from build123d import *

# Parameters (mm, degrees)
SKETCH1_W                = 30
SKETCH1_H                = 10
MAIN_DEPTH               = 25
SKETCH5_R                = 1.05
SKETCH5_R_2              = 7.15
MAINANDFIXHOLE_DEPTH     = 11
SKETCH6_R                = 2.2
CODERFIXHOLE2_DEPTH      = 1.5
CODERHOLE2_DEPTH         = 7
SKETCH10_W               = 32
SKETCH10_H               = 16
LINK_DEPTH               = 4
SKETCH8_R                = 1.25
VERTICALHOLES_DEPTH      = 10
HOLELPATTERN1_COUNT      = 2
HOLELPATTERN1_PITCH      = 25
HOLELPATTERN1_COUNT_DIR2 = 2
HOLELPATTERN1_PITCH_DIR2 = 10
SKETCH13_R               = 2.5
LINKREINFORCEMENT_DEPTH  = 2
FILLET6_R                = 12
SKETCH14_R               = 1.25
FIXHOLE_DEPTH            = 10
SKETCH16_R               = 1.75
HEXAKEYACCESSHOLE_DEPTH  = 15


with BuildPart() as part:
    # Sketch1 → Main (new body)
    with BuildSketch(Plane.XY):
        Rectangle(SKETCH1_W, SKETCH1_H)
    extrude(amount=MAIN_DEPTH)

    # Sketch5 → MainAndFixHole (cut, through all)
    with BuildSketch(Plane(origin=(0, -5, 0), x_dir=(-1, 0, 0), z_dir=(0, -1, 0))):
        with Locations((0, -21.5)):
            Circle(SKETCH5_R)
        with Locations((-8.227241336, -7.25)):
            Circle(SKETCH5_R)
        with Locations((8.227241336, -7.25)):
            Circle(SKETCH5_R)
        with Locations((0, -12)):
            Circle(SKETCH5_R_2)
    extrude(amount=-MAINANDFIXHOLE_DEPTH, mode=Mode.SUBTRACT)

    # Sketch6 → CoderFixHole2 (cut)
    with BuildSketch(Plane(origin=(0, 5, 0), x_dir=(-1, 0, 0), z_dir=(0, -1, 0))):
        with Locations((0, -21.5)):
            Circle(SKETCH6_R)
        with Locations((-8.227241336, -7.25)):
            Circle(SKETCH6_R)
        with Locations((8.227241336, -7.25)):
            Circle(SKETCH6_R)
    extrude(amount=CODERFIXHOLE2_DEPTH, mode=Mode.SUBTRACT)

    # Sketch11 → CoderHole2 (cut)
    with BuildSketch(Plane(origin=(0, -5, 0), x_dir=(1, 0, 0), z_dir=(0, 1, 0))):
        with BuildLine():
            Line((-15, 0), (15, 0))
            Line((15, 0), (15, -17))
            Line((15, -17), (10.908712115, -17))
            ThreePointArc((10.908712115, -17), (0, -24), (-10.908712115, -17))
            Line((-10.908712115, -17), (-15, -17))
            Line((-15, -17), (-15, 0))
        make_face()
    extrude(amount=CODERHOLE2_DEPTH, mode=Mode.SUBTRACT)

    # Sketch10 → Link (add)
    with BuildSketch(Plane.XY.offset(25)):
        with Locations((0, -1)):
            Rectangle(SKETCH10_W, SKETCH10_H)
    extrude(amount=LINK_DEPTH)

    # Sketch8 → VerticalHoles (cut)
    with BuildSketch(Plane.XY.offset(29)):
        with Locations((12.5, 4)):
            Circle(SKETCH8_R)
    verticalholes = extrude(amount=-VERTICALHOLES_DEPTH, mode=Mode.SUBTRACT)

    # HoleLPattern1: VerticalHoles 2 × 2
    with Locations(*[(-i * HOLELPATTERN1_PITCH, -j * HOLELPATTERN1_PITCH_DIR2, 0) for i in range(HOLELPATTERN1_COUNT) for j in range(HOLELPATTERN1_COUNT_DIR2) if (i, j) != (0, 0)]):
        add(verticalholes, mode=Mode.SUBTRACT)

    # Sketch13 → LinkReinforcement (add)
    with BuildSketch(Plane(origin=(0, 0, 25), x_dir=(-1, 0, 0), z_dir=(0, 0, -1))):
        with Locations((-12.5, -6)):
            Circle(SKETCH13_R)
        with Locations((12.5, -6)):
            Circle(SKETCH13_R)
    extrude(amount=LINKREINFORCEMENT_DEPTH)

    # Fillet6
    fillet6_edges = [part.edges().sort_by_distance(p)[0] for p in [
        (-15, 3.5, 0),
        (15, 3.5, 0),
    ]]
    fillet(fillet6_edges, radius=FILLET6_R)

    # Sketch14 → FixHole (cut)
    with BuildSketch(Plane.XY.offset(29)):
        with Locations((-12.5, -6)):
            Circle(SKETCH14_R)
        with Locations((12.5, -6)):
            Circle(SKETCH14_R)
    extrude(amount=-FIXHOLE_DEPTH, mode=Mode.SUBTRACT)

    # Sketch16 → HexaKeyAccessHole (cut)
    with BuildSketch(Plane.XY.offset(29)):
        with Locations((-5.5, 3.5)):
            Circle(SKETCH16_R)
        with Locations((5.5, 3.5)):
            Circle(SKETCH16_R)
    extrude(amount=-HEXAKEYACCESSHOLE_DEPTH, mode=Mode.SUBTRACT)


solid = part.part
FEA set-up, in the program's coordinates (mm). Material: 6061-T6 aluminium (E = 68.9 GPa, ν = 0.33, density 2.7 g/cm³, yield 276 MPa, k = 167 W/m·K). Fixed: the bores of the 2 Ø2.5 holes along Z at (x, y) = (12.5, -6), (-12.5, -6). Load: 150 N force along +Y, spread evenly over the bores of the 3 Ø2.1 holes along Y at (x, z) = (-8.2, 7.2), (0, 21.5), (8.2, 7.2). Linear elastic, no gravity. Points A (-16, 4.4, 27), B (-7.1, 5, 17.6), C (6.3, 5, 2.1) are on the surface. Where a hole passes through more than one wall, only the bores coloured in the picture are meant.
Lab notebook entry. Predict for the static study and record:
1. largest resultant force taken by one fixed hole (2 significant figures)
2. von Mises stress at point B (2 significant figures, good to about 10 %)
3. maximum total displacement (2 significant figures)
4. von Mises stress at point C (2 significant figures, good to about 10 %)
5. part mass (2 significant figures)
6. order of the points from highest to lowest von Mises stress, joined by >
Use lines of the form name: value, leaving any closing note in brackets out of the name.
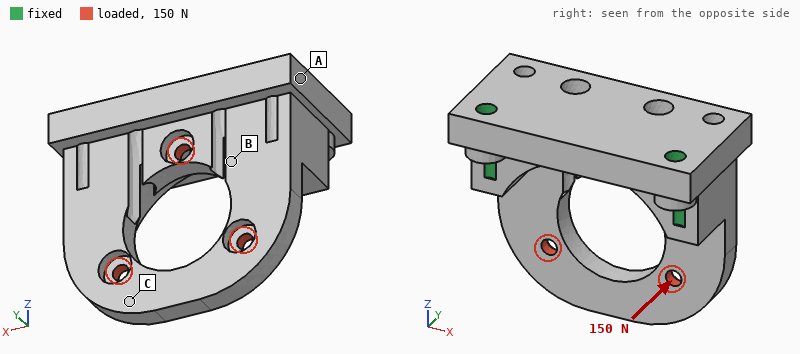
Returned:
largest resultant force taken by one fixed hole: 84 N
von Mises stress at point B: 35 MPa
maximum total displacement: 57 µm
von Mises stress at point C: 8.2 MPa
part mass: 11 g
order of the points from highest to lowest von Mises stress, joined by >: B > C > A
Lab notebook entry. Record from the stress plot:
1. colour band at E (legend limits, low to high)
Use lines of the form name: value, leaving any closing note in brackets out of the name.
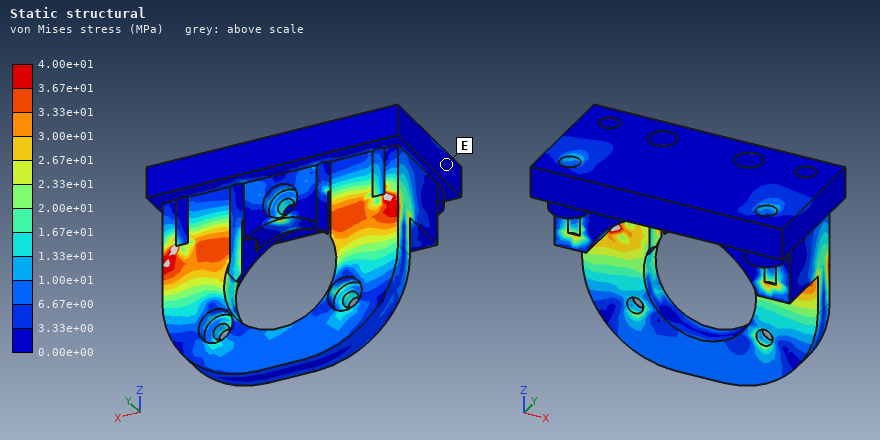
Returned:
colour band at E: 0.00e+00 to 3.33e+00 MPa
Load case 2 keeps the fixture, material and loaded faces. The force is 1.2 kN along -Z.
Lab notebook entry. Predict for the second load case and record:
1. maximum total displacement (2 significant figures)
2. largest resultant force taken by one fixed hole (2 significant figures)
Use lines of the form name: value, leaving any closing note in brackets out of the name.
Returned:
maximum total displacement: 22 µm
largest resultant force taken by one fixed hole: 600 N
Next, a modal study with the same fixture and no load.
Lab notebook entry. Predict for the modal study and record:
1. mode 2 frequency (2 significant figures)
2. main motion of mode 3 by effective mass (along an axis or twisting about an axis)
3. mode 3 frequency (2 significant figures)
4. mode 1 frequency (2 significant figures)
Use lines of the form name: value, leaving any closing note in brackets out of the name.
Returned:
mode 2 frequency: 12 kHz
main motion of mode 3 by effective mass: along X
mode 3 frequency: 14 kHz
mode 1 frequency: 5500 Hz
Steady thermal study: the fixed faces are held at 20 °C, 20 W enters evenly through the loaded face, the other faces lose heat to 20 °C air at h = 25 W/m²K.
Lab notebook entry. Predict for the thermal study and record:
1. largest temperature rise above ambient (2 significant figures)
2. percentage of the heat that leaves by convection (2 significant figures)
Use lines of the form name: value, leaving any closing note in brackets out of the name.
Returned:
largest temperature rise above ambient: 35 K
percentage of the heat that leaves by convection: 4.0 %
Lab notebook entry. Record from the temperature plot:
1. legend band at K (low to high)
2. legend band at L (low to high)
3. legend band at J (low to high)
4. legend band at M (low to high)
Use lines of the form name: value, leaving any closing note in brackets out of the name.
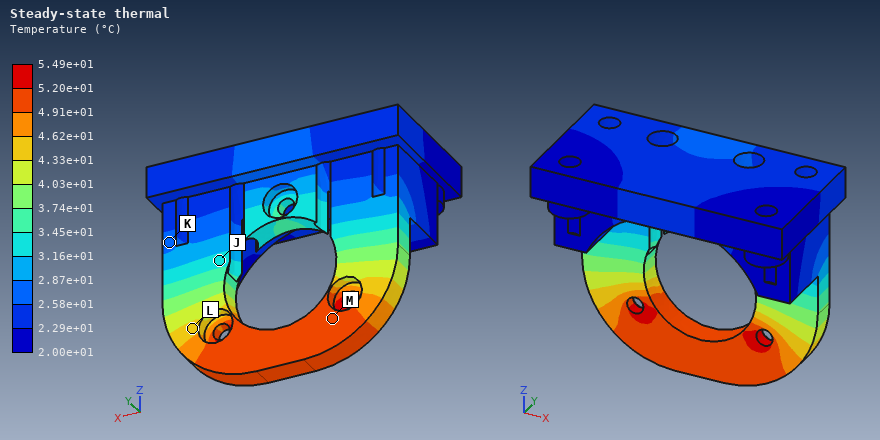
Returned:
legend band at K: 2.58e+01 to 2.87e+01 °C
legend band at L: 4.33e+01 to 4.62e+01 °C
legend band at J: 3.16e+01 to 3.45e+01 °C
legend band at M: 4.91e+01 to 5.20e+01 °C
